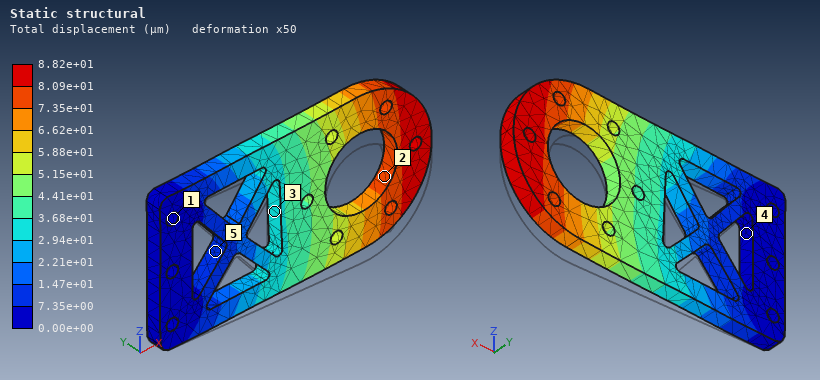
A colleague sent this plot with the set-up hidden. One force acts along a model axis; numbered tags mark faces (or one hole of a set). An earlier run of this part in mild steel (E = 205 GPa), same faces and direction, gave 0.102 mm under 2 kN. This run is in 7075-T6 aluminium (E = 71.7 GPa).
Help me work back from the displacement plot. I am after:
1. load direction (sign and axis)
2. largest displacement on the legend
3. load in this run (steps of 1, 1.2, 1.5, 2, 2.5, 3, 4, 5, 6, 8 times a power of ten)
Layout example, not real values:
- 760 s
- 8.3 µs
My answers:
- +Z
- 8.82e+01 µm
- 600 N
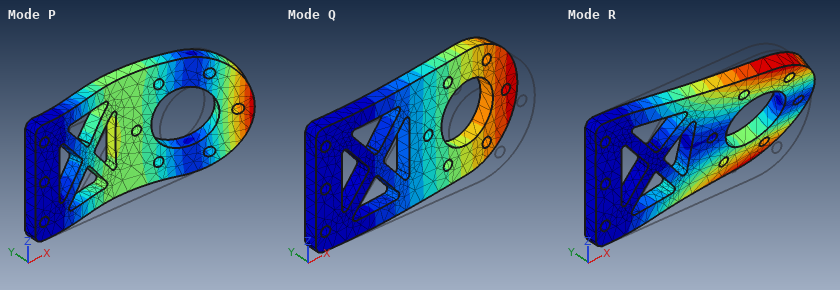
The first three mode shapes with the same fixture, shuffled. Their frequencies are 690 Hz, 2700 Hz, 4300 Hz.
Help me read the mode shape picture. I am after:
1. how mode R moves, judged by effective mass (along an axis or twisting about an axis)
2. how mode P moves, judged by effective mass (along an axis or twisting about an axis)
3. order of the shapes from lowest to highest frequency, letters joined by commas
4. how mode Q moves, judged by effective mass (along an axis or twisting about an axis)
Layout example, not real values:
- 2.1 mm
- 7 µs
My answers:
- twisting about X
- along Y
- Q, R, P
- along Y
